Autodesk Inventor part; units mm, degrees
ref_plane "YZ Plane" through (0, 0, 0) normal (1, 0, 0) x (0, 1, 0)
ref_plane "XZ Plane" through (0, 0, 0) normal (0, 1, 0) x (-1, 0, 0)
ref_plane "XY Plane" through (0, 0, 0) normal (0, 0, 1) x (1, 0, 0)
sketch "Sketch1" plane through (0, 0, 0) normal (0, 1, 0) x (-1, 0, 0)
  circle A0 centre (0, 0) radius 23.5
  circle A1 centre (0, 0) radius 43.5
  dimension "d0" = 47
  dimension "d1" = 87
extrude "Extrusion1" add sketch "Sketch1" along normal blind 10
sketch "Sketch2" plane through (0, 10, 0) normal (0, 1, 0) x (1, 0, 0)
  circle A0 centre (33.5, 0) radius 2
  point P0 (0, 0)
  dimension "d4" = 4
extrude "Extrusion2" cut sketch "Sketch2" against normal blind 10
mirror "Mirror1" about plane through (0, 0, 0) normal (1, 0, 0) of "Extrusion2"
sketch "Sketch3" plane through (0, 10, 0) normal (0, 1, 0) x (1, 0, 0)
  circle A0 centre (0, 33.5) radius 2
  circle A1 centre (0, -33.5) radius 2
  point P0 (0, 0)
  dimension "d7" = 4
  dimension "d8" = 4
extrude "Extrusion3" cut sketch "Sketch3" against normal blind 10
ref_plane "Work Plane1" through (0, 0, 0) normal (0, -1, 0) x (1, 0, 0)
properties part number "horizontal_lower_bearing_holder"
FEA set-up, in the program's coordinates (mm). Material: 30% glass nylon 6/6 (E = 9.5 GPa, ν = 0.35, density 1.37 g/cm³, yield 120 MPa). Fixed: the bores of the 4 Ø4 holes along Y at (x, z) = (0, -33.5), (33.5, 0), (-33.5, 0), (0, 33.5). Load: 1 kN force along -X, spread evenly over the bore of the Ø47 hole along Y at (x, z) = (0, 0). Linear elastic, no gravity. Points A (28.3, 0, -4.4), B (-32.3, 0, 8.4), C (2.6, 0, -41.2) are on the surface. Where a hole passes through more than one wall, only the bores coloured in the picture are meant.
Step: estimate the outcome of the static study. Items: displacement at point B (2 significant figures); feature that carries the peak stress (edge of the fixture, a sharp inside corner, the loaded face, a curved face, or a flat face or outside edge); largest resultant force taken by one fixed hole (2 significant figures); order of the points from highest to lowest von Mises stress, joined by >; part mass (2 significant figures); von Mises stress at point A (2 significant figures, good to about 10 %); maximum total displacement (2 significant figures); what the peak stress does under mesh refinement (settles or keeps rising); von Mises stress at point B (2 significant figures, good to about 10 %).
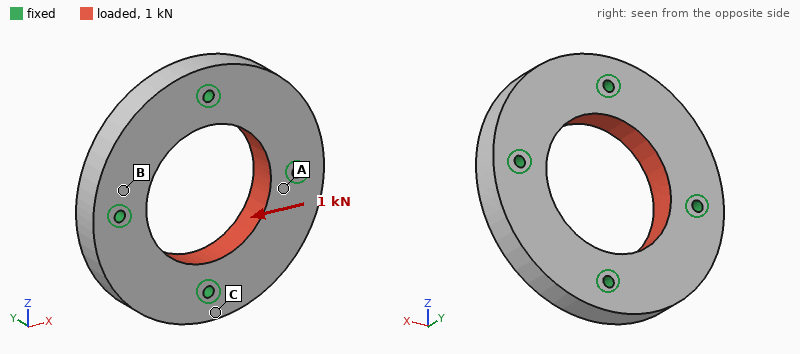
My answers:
1.6 µm
edge of the fixture
280 N
A > B > C
57 g
1.4 MPa
3.8 µm
keeps rising
0.86 MPa
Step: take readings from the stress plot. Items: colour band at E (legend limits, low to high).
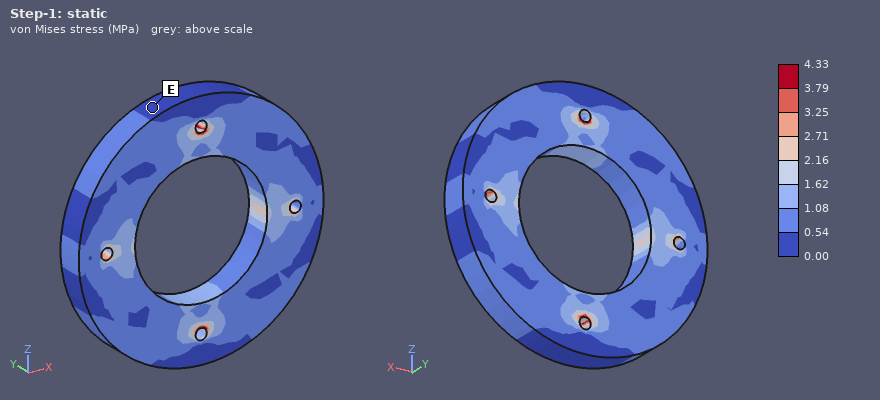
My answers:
0.00 to 0.54 MPa
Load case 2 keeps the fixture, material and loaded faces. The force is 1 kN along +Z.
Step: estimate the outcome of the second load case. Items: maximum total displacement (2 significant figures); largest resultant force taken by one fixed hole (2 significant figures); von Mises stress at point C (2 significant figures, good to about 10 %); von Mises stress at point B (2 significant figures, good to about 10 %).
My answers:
3.8 µm
280 N
0.60 MPa
1.1 MPa
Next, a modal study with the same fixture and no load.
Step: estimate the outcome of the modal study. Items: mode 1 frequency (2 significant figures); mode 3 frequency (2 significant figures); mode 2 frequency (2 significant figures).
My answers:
5800 Hz
6400 Hz
6400 Hz
